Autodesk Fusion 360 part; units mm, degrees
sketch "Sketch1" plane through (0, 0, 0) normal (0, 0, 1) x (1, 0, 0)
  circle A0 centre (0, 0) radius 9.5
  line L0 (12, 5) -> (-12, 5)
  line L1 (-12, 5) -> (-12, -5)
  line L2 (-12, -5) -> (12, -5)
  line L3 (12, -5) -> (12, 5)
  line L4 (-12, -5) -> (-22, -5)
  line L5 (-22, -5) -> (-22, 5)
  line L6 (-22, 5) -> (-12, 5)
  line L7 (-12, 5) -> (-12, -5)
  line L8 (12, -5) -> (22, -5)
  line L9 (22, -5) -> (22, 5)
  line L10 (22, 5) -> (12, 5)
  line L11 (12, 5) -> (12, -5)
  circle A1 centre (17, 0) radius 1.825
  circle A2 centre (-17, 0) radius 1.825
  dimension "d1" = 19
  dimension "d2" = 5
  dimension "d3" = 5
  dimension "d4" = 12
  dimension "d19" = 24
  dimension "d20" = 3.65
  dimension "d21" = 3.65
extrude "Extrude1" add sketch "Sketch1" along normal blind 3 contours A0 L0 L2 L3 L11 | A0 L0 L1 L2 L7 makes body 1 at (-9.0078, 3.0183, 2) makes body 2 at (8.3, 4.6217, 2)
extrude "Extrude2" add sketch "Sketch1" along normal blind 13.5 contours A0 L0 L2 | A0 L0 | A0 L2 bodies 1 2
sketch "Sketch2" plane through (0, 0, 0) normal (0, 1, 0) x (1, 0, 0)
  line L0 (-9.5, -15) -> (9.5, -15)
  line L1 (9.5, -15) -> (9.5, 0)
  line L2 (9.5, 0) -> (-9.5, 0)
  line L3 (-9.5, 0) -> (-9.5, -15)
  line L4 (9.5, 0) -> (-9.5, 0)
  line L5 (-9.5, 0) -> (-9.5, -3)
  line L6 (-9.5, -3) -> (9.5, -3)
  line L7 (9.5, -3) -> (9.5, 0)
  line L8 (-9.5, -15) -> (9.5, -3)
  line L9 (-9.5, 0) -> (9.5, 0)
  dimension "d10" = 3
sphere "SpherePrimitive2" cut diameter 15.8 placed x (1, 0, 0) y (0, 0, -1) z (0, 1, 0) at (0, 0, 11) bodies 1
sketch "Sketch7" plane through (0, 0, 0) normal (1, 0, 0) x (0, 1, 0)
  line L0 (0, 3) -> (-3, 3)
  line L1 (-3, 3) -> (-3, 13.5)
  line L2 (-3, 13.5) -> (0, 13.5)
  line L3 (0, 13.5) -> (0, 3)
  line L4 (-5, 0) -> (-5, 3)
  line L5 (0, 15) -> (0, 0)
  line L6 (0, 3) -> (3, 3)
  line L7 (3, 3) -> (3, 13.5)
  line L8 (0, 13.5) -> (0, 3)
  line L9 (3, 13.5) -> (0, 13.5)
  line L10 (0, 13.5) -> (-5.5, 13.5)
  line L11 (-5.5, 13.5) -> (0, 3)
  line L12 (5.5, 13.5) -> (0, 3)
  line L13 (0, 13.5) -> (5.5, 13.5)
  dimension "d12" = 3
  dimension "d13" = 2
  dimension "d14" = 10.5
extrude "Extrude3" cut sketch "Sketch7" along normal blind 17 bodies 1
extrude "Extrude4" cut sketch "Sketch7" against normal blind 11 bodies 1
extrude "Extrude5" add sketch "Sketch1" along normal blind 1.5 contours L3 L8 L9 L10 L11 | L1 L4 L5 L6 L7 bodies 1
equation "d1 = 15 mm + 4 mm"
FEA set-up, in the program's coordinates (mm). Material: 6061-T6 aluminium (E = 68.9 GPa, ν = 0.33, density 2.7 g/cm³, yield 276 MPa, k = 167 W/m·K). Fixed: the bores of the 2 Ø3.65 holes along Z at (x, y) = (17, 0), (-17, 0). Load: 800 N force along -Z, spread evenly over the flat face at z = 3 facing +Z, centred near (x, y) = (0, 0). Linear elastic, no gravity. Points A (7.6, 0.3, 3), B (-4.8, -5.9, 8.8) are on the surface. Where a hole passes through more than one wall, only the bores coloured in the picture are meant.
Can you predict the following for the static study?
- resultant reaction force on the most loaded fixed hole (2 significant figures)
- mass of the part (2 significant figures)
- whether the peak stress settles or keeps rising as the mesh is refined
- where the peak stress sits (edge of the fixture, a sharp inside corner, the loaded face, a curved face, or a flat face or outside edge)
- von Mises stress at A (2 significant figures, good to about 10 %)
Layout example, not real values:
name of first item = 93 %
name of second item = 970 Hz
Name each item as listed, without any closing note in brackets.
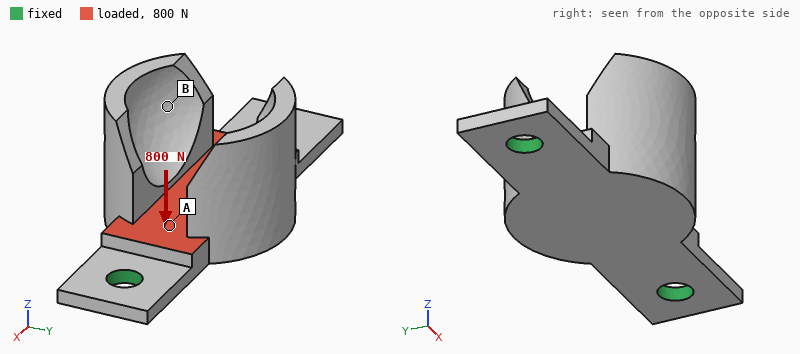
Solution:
resultant reaction force on the most loaded fixed hole = 580 N
mass of the part = 6.3 g
whether the peak stress settles or keeps rising as the mesh is refined = keeps rising
where the peak stress sits = edge of the fixture
von Mises stress at A = 61 MPa
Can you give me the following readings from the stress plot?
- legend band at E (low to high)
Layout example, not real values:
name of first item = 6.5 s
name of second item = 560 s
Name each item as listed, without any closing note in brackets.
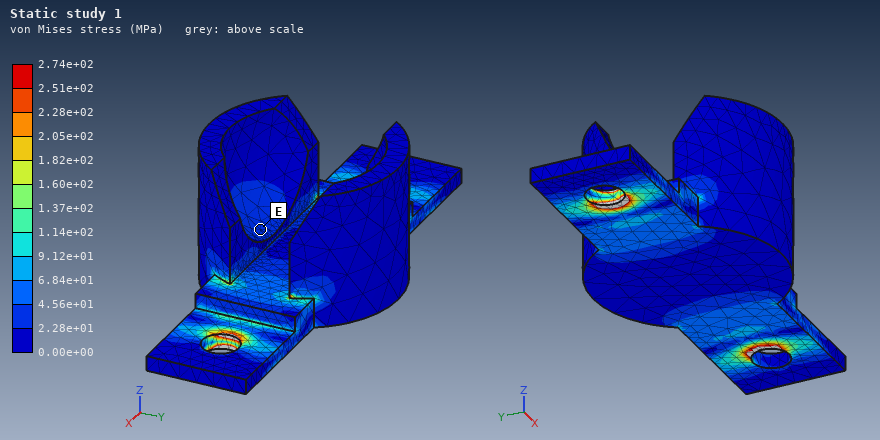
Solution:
legend band at E = 2.28e+01 to 4.56e+01 MPa
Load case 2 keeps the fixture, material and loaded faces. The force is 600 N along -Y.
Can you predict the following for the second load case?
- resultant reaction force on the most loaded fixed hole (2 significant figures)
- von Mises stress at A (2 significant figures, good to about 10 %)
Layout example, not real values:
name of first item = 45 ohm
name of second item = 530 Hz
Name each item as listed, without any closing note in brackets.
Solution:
resultant reaction force on the most loaded fixed hole = 300 N
von Mises stress at A = 29 MPa
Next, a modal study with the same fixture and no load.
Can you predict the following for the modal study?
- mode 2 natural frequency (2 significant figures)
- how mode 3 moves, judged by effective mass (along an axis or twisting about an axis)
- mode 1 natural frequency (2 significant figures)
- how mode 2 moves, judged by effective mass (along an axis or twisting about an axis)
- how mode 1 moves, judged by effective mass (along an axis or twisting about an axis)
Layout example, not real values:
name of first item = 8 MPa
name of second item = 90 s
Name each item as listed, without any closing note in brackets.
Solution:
mode 2 natural frequency = 7900 Hz
how mode 3 moves, judged by effective mass = along X
mode 1 natural frequency = 3700 Hz
how mode 2 moves, judged by effective mass = along Z
how mode 1 moves, judged by effective mass = along Y
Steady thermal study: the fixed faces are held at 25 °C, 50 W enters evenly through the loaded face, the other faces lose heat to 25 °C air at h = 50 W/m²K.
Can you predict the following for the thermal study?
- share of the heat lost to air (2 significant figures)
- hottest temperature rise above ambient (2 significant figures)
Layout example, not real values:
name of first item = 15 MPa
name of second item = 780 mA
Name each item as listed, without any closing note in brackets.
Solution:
share of the heat lost to air = 9.4 %
hottest temperature rise above ambient = 66 K
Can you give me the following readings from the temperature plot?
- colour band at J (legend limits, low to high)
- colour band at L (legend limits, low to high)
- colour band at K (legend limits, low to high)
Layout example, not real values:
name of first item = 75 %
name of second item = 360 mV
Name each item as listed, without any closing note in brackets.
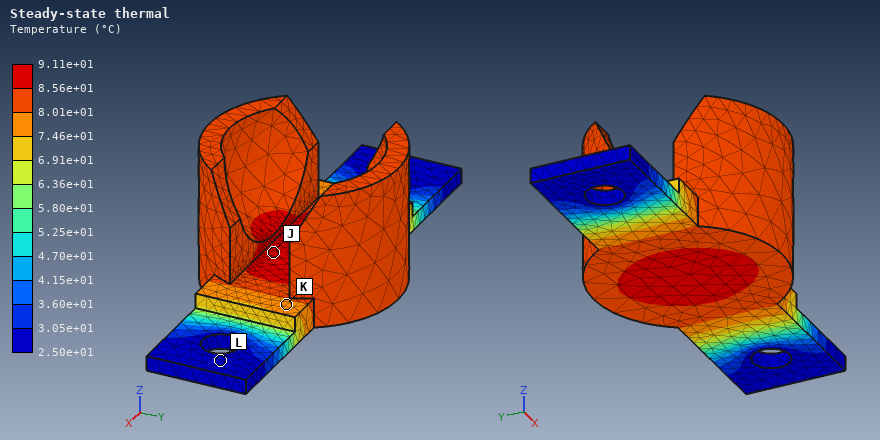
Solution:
colour band at J = 8.56e+01 to 9.11e+01 °C
colour band at L = 2.50e+01 to 3.05e+01 °C
colour band at K = 7.46e+01 to 8.01e+01 °C
